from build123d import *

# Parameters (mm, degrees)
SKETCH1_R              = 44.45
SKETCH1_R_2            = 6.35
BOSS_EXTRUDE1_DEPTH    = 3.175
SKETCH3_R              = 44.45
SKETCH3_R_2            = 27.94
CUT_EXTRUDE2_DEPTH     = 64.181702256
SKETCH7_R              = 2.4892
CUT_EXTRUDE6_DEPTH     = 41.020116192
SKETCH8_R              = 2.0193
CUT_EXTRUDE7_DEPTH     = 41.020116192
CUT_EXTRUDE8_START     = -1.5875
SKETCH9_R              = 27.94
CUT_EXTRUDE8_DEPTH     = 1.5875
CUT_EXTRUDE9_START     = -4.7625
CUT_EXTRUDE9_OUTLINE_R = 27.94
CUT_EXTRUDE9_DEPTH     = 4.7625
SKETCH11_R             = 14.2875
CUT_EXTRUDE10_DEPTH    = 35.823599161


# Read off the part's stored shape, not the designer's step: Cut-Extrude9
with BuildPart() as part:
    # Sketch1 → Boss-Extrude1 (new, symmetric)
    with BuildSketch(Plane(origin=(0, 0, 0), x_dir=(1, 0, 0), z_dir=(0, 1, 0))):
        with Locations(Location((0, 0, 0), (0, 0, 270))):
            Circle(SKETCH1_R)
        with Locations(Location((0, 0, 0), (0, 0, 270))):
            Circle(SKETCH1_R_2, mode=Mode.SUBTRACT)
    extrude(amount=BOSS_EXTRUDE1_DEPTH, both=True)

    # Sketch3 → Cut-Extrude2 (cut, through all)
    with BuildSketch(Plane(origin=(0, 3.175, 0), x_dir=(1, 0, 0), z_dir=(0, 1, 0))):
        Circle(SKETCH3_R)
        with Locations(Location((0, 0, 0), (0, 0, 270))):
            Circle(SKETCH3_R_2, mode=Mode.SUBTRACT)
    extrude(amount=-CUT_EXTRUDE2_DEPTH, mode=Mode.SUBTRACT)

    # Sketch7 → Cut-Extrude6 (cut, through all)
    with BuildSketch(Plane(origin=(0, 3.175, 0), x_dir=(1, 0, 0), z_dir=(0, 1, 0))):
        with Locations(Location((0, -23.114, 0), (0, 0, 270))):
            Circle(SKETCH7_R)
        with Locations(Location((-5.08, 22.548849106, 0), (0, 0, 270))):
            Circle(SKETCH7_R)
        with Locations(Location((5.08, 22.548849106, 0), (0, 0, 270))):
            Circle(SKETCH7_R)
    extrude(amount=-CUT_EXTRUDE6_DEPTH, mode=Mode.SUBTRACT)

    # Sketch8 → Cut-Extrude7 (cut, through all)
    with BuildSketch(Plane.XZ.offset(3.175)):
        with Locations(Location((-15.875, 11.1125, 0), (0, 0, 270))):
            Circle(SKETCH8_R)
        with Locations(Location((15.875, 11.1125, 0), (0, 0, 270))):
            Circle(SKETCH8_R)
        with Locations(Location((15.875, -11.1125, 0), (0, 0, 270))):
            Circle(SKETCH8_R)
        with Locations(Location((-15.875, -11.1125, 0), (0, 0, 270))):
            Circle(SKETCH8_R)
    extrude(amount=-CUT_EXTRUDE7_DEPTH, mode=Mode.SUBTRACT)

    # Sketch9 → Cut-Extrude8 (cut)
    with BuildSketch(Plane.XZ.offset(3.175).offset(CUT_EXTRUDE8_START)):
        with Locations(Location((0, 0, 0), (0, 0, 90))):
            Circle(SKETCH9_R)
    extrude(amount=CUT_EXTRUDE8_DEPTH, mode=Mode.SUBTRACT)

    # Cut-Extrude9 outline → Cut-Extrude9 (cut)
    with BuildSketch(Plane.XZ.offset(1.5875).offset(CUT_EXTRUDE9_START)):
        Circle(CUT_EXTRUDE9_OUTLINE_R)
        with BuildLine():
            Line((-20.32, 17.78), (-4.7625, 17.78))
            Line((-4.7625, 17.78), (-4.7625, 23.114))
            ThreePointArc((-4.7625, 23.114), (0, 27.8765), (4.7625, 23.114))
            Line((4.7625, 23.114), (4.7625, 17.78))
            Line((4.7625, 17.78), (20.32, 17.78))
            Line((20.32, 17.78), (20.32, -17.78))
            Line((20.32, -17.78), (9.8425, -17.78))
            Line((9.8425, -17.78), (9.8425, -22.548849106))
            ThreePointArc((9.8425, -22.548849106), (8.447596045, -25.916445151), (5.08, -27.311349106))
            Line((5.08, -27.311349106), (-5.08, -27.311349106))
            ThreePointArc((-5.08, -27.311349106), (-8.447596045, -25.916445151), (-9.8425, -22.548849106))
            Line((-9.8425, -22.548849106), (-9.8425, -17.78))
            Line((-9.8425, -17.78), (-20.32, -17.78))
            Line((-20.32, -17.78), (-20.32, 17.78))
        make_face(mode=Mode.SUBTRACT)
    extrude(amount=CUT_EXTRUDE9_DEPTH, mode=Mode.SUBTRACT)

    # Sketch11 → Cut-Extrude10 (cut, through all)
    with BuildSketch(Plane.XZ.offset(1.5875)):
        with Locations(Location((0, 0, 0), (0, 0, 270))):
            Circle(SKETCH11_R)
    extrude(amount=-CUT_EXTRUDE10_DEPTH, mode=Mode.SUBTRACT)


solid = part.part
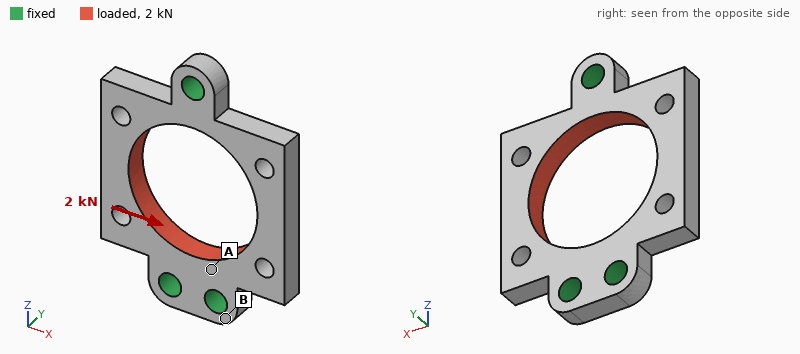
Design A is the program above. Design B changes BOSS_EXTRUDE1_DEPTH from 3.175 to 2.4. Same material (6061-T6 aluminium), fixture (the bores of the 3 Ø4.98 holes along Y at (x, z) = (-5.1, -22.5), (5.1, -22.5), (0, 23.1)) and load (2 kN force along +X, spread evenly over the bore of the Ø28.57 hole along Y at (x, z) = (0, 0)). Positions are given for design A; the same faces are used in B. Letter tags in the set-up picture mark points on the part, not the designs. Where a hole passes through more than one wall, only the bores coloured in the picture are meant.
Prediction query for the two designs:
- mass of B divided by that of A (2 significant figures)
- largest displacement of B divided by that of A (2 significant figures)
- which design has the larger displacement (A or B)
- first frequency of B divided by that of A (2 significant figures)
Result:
0.84
1.2
B
0.87
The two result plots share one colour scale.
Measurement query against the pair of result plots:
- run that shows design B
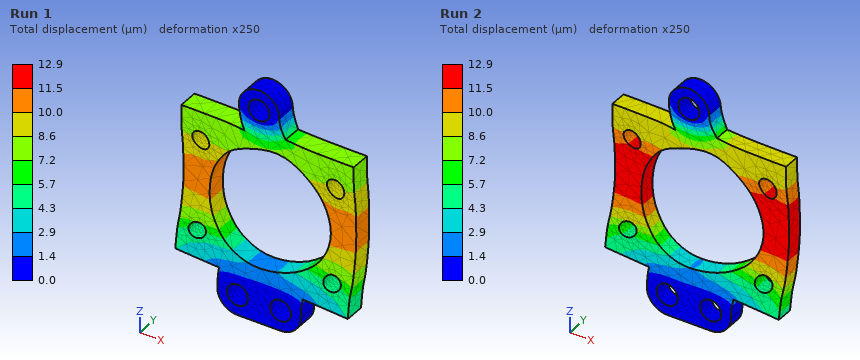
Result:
Run 2
